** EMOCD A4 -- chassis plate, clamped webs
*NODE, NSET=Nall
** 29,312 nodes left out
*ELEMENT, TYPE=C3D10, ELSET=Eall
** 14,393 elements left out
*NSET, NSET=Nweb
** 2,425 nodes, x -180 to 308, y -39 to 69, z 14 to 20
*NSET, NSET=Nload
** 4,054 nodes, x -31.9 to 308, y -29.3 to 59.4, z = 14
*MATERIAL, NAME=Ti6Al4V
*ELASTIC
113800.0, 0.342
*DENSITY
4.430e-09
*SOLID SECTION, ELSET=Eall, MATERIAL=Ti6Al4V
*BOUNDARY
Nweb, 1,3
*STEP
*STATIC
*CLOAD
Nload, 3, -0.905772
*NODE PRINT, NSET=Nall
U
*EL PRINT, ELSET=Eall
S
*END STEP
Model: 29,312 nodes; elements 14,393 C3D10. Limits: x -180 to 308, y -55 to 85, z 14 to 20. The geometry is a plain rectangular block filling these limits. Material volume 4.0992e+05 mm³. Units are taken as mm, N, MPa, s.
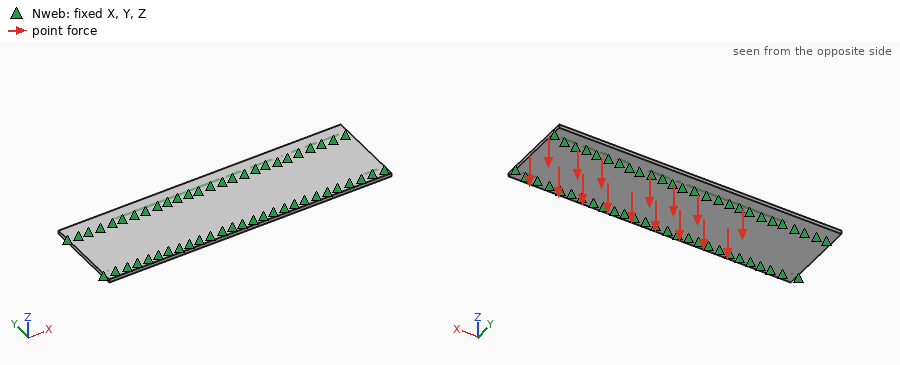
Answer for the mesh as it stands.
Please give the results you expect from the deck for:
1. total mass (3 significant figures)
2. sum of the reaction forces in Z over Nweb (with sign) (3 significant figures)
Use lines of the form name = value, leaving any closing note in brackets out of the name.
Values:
total mass = 1.82 kg
sum of the reaction forces in Z over Nweb (with sign) = 3670 N
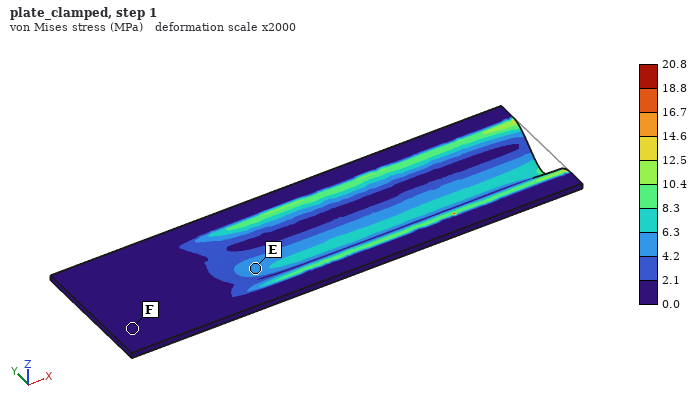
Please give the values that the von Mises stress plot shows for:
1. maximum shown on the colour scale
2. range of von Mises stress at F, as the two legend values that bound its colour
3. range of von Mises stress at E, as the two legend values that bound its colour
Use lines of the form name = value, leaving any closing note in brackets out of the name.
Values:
maximum shown on the colour scale = 20.8 MPa
range of von Mises stress at F, as the two legend values that bound its colour = 0.0 to 2.1 MPa
range of von Mises stress at E, as the two legend values that bound its colour = 4.2 to 6.3 MPa
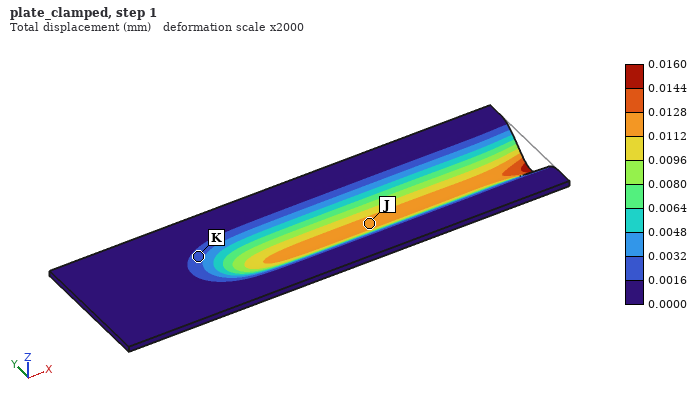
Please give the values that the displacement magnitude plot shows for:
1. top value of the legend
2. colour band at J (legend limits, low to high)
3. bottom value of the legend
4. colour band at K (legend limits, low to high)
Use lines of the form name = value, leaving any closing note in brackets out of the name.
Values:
top value of the legend = 0.0160 mm
colour band at J = 0.0112 to 0.0128 mm
bottom value of the legend = 0.0000 mm
colour band at K = 0.0016 to 0.0032 mm
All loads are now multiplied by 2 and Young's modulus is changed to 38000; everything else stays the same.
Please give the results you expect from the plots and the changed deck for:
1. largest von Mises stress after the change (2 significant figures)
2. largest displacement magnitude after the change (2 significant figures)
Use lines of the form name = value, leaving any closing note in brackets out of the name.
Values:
largest von Mises stress after the change = 42 MPa
largest displacement magnitude after the change = 0.096 mm
